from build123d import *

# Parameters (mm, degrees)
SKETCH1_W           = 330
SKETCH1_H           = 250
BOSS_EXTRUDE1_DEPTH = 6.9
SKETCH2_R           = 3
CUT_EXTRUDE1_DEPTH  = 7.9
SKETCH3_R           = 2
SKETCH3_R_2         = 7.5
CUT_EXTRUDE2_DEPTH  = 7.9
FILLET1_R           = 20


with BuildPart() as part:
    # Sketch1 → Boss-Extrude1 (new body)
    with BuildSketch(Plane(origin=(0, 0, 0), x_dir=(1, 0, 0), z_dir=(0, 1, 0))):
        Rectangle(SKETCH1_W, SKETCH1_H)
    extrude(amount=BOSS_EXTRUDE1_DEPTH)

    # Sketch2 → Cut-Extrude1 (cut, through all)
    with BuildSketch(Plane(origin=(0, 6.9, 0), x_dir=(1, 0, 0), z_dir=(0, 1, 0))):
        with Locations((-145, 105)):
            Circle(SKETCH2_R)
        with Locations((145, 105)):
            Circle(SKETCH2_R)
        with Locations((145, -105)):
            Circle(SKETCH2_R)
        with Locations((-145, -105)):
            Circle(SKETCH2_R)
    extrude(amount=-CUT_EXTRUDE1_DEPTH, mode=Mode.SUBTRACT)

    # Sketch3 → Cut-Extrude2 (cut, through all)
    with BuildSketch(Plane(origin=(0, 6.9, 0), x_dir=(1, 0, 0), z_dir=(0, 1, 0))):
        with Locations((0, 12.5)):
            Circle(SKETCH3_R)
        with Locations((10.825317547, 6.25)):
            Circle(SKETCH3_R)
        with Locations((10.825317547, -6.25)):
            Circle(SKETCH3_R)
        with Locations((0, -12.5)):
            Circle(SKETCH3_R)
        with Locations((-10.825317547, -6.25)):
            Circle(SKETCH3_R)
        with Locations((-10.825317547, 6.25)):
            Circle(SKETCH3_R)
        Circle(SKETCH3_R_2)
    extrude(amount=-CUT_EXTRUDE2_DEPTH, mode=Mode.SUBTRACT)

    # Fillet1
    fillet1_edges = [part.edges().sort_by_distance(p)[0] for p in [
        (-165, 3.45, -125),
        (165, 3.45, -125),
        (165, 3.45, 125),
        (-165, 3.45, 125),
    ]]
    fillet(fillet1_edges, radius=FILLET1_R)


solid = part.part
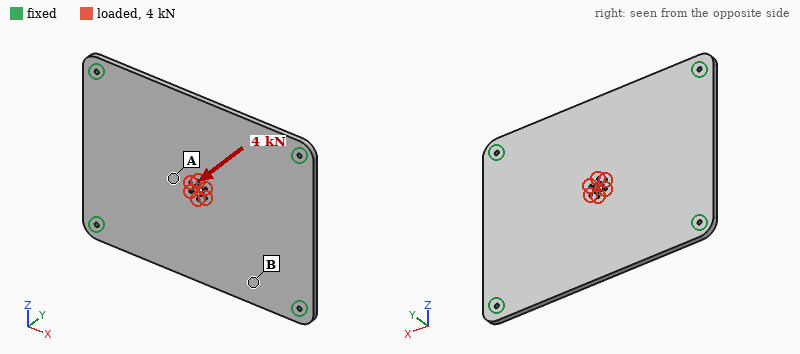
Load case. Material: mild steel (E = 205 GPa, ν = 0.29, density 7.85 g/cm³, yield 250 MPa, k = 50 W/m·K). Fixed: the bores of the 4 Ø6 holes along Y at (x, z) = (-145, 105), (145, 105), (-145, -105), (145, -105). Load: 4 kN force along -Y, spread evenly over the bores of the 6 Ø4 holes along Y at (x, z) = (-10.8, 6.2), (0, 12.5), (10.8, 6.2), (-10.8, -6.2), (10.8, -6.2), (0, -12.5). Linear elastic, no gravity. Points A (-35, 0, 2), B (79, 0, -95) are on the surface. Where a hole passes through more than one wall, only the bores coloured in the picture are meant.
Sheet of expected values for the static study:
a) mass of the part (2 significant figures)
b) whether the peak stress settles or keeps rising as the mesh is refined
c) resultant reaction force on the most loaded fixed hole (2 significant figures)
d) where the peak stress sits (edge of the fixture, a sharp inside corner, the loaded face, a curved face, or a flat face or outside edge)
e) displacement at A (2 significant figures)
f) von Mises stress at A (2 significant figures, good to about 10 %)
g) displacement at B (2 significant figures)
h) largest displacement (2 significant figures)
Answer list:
4.4 kg
keeps rising
1.0 kN
edge of the fixture
0.68 mm
77 MPa
0.26 mm
0.79 mm
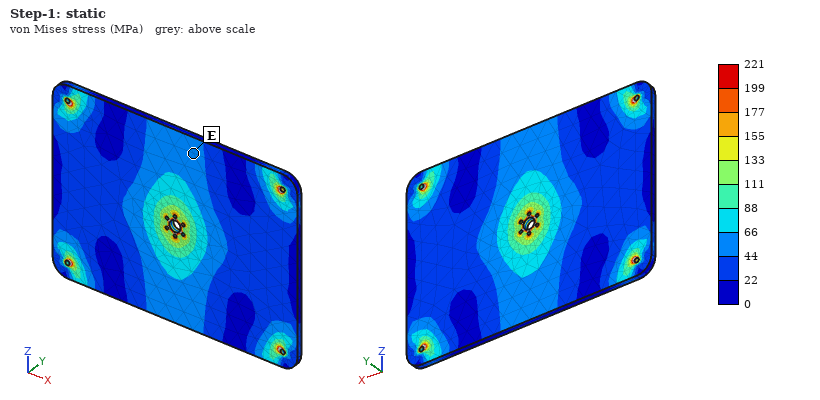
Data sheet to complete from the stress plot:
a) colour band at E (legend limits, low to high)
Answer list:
44 to 66 MPa
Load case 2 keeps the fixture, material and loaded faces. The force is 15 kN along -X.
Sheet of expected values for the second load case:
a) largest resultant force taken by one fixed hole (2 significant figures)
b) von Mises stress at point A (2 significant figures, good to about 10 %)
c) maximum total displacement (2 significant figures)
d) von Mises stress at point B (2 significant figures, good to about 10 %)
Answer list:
4.0 kN
16 MPa
12 µm
6.5 MPa
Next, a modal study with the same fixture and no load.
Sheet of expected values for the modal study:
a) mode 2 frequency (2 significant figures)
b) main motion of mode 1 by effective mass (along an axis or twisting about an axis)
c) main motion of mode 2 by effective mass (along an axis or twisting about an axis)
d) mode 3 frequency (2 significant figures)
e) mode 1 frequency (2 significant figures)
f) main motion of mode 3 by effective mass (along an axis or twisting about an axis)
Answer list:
510 Hz
along Y
twisting about X
720 Hz
320 Hz
twisting about Z
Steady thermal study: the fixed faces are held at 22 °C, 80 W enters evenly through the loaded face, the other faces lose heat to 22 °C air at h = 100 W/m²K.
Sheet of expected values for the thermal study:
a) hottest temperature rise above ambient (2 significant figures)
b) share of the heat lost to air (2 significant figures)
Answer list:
58 K
98 %
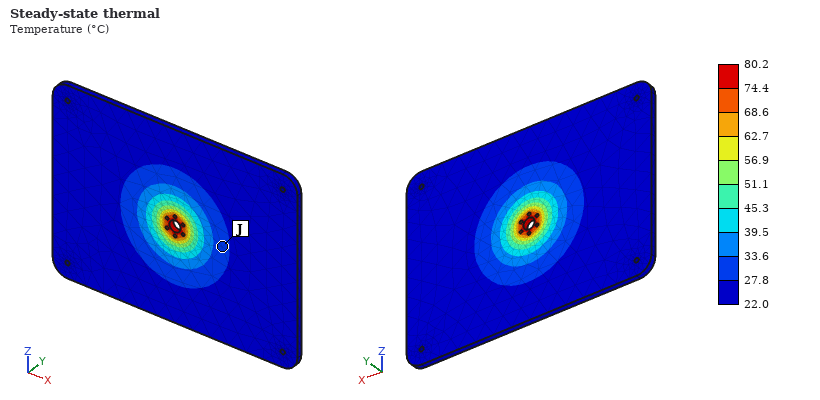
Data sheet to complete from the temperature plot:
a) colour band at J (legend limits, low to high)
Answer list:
27.8 to 33.6 °C
